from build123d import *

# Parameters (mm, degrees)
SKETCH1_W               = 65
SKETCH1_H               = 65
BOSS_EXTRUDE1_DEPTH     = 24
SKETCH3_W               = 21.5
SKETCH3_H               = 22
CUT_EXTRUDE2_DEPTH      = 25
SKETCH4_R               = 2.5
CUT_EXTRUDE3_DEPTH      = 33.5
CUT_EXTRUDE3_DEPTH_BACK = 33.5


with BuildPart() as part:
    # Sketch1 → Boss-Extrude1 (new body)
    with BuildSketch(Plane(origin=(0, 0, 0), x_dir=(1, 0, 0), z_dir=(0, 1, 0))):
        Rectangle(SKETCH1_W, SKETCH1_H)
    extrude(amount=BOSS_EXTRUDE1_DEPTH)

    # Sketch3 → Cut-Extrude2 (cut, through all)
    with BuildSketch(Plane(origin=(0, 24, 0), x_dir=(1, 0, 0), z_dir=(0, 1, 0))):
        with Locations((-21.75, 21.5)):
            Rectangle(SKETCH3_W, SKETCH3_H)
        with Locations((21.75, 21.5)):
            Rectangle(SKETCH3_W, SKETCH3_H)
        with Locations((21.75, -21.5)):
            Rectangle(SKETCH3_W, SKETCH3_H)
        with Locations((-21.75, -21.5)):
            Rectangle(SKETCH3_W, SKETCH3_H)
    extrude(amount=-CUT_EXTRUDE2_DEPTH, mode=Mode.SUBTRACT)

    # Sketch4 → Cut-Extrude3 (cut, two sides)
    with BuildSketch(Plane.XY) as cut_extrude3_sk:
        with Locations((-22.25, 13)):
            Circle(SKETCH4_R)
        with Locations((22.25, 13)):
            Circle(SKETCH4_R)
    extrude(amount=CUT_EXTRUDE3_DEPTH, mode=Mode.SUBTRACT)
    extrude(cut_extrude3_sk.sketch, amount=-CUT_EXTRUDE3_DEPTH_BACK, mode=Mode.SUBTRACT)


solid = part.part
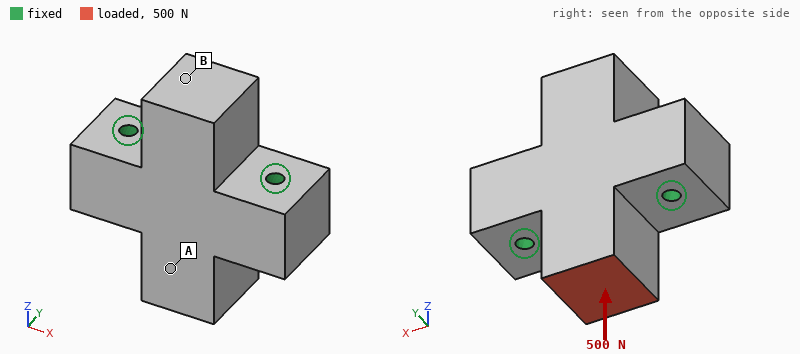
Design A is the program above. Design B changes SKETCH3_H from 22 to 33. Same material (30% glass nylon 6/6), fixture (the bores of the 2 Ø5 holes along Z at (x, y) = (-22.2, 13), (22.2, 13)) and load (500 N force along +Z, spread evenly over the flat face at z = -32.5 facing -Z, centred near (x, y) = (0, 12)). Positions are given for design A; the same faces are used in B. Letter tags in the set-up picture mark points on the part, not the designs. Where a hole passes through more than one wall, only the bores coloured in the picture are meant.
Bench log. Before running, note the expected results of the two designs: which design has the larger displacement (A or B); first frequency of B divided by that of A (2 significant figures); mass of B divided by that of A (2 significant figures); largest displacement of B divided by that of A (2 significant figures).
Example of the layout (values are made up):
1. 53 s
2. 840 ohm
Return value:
1. B
2. 0.49
3. 0.80
4. 2.2
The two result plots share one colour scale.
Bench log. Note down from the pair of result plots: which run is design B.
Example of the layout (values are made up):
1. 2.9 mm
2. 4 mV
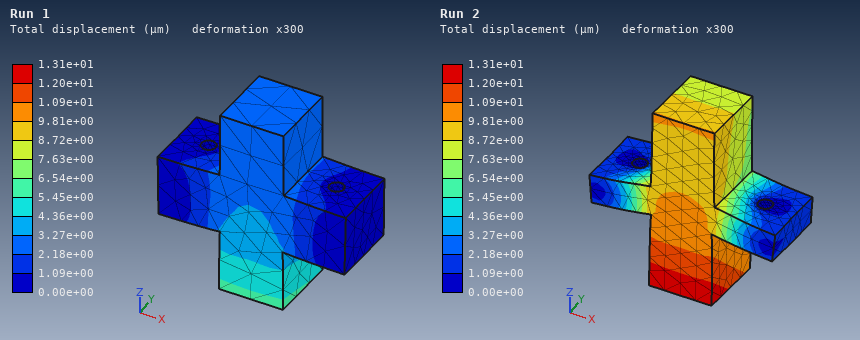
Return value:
1. Run 2
